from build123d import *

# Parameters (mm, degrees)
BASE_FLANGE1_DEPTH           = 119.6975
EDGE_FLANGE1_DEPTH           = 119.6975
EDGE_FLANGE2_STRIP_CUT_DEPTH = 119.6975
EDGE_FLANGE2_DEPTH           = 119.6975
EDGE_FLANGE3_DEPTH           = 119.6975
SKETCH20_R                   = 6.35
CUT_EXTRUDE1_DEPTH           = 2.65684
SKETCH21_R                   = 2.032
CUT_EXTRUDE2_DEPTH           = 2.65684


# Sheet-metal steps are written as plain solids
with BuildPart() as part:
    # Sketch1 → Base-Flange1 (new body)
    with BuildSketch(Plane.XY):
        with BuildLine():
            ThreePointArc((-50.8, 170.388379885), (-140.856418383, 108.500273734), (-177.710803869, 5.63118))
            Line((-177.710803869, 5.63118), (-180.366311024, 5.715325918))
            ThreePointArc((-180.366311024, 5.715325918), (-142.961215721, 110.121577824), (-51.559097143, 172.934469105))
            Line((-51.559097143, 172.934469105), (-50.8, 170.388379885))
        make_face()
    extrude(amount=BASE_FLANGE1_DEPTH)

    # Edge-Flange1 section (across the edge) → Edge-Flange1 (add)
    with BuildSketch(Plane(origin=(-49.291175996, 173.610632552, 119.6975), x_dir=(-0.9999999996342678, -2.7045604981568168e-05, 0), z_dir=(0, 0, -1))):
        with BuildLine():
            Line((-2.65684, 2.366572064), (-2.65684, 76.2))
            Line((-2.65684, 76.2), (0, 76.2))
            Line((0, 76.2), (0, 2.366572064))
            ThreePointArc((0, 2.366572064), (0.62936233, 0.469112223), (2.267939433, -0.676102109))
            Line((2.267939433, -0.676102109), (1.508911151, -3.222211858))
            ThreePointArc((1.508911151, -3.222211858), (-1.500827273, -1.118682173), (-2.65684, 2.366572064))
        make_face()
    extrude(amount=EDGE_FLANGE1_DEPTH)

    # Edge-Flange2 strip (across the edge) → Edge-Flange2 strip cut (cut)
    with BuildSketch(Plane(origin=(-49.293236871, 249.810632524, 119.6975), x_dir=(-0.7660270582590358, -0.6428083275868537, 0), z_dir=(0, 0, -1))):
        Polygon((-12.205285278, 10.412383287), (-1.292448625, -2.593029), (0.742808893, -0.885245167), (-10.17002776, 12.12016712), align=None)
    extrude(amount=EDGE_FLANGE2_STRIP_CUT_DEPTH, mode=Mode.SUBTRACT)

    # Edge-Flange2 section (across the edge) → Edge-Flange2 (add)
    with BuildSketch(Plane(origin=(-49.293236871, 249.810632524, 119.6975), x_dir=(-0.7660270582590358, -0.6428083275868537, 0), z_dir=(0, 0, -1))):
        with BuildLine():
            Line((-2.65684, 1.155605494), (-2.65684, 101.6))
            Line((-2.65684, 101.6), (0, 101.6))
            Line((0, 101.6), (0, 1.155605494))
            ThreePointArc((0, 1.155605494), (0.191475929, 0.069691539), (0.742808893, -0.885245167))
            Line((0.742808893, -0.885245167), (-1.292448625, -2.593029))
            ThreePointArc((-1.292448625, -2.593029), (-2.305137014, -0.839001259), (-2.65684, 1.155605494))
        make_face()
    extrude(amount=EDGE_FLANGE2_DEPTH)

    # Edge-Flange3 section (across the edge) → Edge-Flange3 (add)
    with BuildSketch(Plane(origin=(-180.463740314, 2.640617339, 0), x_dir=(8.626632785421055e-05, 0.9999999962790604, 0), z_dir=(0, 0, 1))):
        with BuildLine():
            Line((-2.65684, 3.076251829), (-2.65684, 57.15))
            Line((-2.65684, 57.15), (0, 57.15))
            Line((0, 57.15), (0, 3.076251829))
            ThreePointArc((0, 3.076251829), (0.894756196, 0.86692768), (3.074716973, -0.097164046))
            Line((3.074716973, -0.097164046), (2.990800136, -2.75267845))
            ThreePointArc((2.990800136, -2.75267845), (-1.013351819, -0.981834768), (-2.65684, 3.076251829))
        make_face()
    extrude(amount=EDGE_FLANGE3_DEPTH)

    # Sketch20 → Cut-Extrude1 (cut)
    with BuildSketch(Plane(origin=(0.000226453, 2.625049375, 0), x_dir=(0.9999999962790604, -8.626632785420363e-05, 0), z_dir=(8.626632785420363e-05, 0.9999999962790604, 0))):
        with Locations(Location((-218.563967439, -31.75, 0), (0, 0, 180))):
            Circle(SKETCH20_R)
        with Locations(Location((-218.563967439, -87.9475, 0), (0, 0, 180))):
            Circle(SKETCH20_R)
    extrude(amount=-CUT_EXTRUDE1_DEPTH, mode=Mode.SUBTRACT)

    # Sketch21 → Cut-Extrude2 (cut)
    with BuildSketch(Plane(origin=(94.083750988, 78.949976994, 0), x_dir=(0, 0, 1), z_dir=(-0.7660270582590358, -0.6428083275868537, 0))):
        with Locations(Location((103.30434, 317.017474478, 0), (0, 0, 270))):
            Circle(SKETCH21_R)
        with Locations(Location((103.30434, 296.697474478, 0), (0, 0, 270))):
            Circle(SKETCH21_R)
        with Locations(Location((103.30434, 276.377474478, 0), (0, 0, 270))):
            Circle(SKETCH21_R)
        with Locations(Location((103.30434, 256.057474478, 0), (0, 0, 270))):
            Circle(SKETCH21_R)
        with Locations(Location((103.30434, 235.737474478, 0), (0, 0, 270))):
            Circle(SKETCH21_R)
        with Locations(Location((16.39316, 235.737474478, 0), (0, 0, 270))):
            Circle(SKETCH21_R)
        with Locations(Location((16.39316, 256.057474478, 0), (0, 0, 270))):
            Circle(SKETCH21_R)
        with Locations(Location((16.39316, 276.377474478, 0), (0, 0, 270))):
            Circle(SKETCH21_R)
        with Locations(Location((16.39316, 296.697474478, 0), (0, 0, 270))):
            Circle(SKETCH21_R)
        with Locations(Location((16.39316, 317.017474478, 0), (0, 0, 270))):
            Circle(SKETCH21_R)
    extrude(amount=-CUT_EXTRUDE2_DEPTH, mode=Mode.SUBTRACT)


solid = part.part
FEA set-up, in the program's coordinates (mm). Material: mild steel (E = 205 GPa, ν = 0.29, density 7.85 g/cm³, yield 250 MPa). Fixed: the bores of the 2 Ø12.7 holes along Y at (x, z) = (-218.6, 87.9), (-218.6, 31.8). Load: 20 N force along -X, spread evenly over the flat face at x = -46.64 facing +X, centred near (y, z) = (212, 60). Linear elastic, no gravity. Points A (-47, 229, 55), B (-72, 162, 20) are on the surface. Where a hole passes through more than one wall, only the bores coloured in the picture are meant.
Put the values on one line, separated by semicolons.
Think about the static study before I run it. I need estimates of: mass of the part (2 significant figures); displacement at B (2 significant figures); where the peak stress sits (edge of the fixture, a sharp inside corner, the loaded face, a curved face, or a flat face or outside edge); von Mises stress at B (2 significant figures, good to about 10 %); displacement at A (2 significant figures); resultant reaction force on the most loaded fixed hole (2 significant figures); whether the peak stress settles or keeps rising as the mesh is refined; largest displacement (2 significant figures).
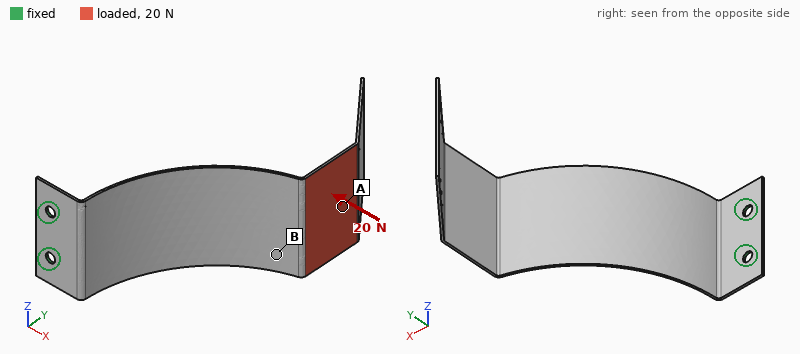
1.2 kg; 2.2 mm; edge of the fixture; 6.4 MPa; 3.3 mm; 12 N; keeps rising; 4.5 mm
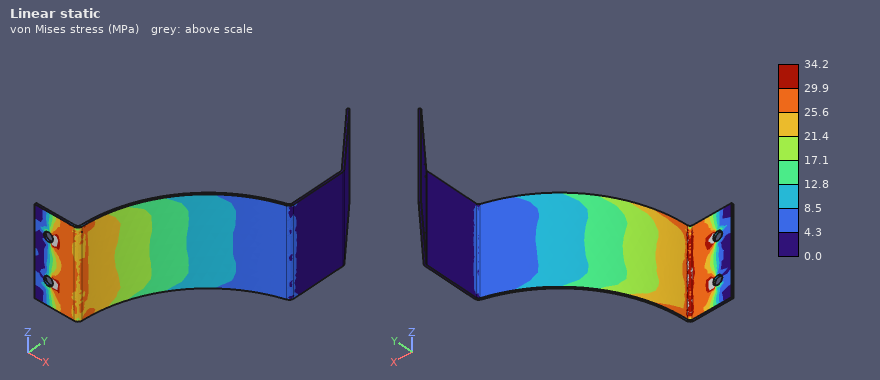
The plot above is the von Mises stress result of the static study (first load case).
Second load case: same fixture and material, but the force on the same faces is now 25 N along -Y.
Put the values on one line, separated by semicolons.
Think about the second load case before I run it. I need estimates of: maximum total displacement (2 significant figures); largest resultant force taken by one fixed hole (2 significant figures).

4.2 mm; 14 N
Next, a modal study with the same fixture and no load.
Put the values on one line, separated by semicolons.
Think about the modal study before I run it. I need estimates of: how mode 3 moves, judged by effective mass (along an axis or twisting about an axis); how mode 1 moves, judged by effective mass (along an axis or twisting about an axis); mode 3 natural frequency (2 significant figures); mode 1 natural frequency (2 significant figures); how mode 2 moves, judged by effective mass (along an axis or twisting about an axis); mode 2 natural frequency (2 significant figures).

along Y; along X; 67 Hz; 13 Hz; along Z; 48 Hz
